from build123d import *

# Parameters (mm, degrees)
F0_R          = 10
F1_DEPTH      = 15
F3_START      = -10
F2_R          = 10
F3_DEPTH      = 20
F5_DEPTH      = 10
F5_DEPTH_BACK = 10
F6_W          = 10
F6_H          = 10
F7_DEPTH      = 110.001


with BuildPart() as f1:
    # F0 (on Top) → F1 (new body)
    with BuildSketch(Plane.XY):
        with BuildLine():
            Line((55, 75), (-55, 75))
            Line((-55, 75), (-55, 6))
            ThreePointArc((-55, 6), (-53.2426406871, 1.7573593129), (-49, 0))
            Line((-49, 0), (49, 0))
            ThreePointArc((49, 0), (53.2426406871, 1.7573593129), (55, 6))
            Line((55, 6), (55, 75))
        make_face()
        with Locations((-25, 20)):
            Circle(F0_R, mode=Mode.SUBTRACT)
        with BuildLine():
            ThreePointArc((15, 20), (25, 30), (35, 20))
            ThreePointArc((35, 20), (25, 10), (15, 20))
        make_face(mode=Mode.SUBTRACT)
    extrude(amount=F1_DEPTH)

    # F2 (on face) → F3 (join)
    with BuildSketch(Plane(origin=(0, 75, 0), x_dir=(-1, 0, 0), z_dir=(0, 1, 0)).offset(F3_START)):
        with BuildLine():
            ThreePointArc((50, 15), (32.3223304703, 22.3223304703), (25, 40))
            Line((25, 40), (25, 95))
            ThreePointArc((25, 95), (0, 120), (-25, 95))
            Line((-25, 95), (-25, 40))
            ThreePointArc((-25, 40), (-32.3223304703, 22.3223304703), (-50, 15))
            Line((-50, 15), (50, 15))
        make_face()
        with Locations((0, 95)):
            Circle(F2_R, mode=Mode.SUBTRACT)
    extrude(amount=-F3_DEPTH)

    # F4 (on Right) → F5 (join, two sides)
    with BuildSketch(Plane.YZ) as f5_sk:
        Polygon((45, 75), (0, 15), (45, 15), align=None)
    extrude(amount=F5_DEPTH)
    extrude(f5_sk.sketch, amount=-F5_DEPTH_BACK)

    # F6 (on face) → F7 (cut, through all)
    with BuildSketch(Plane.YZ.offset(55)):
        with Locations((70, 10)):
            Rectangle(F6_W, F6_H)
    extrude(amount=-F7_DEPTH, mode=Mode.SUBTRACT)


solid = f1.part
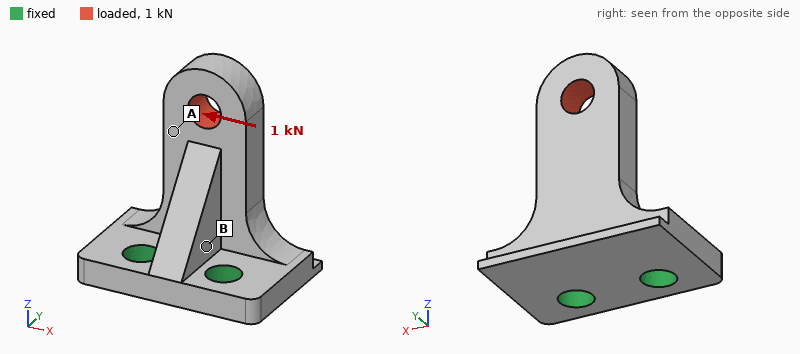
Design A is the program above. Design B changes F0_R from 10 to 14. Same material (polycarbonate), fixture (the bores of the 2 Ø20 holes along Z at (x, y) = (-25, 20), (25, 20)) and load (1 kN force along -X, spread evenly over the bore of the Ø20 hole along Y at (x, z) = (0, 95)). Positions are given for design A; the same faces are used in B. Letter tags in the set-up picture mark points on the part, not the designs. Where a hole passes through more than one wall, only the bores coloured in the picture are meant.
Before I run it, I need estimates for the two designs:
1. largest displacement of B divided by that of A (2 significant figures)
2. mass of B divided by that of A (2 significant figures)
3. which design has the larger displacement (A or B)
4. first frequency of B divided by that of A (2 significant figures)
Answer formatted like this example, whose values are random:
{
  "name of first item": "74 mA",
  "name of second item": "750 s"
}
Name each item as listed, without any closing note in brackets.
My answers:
{
  "largest displacement of B divided by that of A": "0.92",
  "mass of B divided by that of A": "0.98",
  "which design has the larger displacement": "A",
  "first frequency of B divided by that of A": "1.1"
}
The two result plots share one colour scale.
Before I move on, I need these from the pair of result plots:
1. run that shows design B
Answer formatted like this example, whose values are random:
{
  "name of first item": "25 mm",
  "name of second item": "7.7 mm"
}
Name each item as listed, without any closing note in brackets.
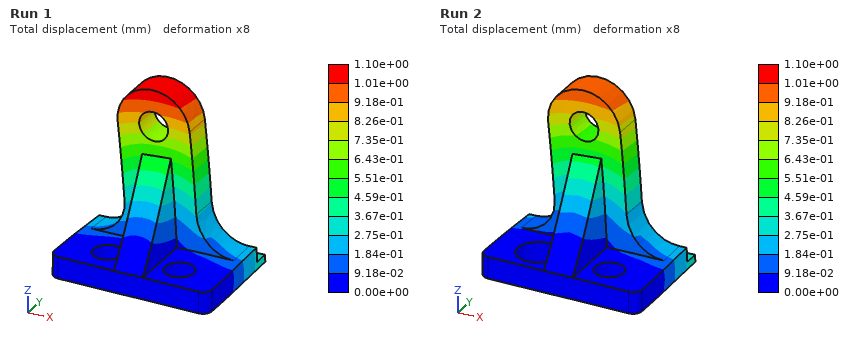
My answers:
{
  "run that shows design B": "Run 2"
}
